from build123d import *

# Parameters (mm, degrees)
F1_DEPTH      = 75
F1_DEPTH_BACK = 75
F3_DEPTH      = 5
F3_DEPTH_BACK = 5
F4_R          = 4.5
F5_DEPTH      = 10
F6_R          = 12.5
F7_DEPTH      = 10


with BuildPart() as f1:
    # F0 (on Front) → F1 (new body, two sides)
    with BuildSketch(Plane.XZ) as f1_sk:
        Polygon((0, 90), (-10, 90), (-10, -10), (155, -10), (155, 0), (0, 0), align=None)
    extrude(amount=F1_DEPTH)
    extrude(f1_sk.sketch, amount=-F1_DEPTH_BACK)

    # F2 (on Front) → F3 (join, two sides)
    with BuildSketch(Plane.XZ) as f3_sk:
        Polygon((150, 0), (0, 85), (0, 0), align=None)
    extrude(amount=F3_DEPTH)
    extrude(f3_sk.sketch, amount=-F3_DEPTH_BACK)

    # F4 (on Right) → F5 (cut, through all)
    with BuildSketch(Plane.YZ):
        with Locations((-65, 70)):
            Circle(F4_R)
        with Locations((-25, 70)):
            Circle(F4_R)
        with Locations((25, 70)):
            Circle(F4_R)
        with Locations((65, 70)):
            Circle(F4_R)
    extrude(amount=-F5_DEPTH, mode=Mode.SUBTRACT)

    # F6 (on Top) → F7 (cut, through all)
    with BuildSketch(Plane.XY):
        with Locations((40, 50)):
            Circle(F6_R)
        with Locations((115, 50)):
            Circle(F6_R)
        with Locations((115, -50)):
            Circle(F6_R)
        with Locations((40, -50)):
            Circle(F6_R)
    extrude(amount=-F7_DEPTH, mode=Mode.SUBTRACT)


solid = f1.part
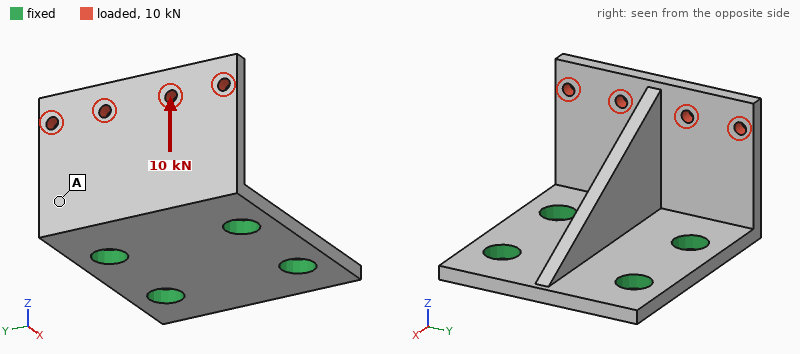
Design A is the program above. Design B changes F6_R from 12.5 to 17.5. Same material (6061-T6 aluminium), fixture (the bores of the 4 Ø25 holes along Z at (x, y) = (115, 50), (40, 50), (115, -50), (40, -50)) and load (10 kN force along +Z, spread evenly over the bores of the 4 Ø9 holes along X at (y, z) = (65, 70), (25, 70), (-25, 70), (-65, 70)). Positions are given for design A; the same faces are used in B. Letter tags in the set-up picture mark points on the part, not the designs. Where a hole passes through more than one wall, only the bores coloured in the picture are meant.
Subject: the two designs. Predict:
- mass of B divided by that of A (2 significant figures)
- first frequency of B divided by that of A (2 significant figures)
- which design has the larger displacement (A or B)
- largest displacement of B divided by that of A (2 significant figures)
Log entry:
0.96
1.1
A
0.71
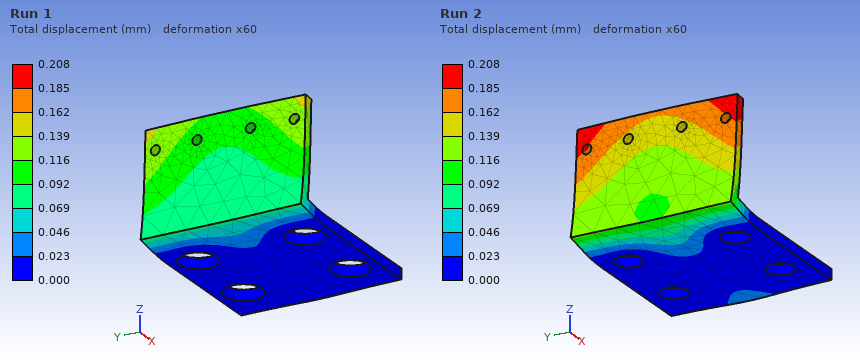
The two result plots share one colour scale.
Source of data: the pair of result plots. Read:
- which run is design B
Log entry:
Run 1
